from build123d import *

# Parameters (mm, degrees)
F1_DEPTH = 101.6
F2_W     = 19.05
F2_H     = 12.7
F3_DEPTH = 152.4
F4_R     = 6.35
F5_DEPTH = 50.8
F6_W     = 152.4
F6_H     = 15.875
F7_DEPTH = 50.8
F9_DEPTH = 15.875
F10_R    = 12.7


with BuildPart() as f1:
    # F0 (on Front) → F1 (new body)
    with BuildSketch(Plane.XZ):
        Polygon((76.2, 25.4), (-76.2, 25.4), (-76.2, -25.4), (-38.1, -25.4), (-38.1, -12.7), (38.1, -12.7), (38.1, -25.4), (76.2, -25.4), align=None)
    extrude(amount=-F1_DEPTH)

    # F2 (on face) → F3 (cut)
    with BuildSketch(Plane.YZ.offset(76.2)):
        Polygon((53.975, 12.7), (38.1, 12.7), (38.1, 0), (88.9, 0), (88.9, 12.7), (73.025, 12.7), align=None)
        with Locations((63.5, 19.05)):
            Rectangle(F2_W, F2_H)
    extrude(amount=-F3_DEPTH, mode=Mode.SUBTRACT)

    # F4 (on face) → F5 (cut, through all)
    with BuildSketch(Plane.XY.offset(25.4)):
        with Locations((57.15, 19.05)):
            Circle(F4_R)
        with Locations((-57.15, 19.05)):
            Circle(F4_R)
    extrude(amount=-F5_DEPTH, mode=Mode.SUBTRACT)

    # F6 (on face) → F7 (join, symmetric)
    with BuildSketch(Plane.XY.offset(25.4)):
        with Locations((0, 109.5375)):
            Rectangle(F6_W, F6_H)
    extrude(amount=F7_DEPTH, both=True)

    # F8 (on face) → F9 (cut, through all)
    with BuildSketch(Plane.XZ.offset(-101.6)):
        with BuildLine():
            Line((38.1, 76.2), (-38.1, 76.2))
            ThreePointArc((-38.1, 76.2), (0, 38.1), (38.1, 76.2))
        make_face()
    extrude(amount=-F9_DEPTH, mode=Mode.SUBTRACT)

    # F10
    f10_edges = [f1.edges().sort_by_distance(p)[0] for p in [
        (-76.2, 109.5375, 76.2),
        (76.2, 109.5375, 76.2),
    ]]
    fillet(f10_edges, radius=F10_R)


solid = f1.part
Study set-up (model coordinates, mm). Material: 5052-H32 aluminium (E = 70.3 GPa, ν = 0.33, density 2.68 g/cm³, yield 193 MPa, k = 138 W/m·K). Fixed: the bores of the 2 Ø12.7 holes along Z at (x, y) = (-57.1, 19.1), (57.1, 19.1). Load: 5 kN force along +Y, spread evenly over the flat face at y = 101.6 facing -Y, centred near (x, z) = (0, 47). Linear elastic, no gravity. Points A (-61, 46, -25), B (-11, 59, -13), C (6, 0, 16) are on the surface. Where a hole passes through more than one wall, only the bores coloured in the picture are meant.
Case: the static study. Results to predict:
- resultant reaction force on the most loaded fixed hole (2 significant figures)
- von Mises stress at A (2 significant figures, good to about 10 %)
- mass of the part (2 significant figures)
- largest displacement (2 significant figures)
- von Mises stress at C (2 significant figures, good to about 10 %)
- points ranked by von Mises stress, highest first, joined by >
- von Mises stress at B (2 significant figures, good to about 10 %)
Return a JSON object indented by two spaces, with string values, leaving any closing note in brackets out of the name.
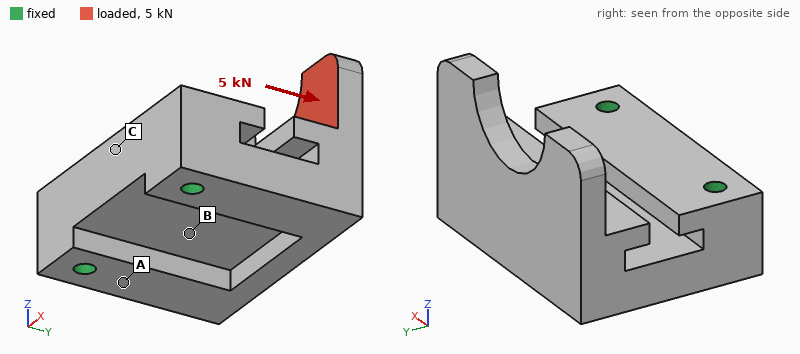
{
  "resultant reaction force on the most loaded fixed hole": "2.9 kN",
  "von Mises stress at A": "27 MPa",
  "mass of the part": "2.0 kg",
  "largest displacement": "0.28 mm",
  "von Mises stress at C": "3.2 MPa",
  "points ranked by von Mises stress, highest first, joined by >": "A > B > C",
  "von Mises stress at B": "12 MPa"
}
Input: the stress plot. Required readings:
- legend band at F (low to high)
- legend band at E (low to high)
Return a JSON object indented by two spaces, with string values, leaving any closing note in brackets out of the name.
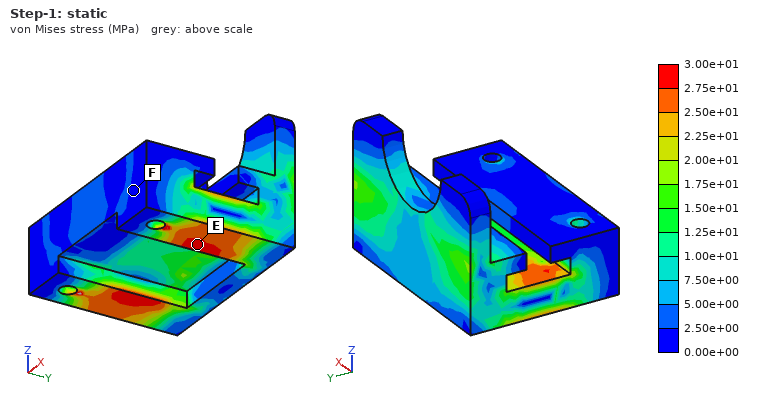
{
  "legend band at F": "0.00e+00 to 2.50e+00 MPa",
  "legend band at E": "2.75e+01 to 3.00e+01 MPa"
}
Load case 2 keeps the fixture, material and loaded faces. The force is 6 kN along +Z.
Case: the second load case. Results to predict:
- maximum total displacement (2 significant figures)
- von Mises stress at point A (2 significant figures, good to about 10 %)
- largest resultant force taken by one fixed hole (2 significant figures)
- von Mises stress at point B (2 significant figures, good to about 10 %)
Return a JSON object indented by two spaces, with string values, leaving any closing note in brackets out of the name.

{
  "maximum total displacement": "0.18 mm",
  "von Mises stress at point A": "33 MPa",
  "largest resultant force taken by one fixed hole": "3.1 kN",
  "von Mises stress at point B": "11 MPa"
}
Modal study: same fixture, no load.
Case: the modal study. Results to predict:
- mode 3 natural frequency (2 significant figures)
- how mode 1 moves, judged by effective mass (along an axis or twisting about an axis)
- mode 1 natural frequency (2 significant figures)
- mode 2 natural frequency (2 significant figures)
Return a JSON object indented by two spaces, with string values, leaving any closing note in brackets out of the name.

{
  "mode 3 natural frequency": "3000 Hz",
  "how mode 1 moves, judged by effective mass": "along Z",
  "mode 1 natural frequency": "1000 Hz",
  "mode 2 natural frequency": "1900 Hz"
}
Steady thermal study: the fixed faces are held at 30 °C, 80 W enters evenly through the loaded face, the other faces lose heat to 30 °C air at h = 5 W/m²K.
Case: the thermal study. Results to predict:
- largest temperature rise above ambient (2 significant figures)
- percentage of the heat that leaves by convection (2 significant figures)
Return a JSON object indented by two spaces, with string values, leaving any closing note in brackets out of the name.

{
  "largest temperature rise above ambient": "27 K",
  "percentage of the heat that leaves by convection": "5.4 %"
}
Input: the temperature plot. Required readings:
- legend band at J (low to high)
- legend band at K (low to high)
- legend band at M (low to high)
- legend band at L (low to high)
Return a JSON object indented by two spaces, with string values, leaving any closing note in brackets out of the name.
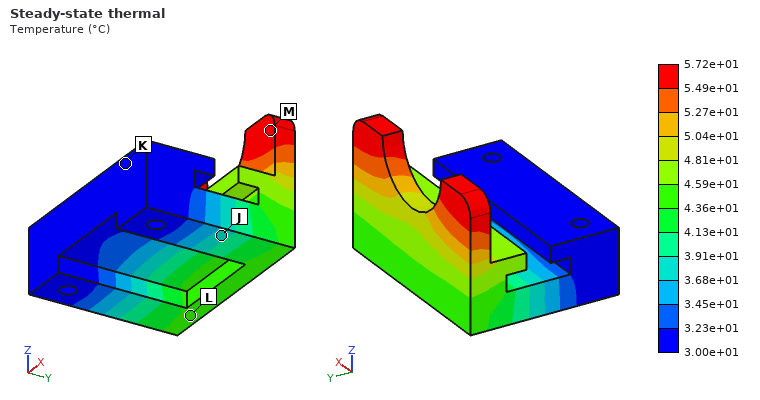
{
  "legend band at J": "3.68e+01 to 3.91e+01 °C",
  "legend band at K": "3.00e+01 to 3.23e+01 °C",
  "legend band at M": "5.49e+01 to 5.72e+01 °C",
  "legend band at L": "4.36e+01 to 4.59e+01 °C"
}
